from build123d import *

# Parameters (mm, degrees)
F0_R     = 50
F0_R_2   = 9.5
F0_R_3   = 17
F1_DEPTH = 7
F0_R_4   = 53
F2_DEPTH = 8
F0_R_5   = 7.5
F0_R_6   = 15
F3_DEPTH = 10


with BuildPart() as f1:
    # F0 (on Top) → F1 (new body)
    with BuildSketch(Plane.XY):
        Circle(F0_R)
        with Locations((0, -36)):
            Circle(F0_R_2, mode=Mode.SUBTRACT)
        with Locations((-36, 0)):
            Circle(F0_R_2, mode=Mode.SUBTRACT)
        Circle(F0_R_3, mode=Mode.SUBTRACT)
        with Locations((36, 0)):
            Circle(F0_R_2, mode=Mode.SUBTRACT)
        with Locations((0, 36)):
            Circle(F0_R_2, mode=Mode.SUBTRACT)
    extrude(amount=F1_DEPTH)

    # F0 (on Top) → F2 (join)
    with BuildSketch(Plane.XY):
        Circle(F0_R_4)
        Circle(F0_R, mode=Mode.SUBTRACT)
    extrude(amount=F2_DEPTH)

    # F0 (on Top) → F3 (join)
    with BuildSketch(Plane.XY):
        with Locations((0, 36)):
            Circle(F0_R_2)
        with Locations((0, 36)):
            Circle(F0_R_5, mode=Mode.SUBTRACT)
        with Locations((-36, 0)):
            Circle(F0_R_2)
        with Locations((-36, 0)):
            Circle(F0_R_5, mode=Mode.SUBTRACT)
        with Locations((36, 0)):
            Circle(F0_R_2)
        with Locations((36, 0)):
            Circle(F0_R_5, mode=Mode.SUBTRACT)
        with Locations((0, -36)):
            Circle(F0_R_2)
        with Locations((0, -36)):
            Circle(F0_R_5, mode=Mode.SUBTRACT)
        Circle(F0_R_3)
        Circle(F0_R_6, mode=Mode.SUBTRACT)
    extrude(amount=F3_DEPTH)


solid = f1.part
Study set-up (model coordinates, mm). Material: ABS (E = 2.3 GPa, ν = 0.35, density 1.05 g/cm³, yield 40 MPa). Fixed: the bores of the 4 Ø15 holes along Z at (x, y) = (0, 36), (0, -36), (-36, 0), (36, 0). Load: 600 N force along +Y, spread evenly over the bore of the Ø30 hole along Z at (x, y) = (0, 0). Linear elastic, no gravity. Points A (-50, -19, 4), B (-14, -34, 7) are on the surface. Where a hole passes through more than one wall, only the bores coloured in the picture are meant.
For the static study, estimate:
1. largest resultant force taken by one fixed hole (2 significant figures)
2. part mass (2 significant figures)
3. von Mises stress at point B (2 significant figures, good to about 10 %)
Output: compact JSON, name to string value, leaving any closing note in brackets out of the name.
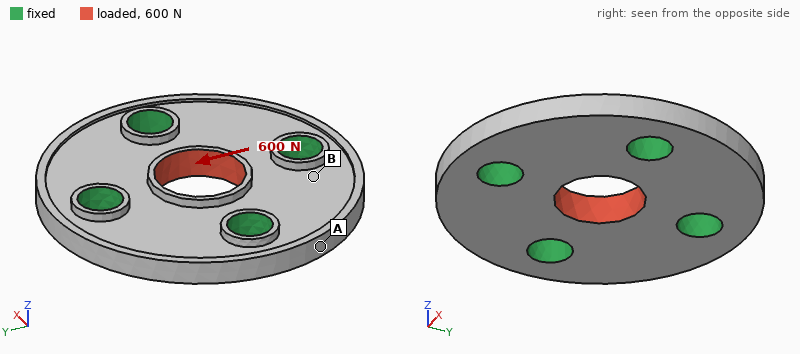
{"largest resultant force taken by one fixed hole": "190 N", "part mass": "57 g", "von Mises stress at point B": "0.41 MPa"}
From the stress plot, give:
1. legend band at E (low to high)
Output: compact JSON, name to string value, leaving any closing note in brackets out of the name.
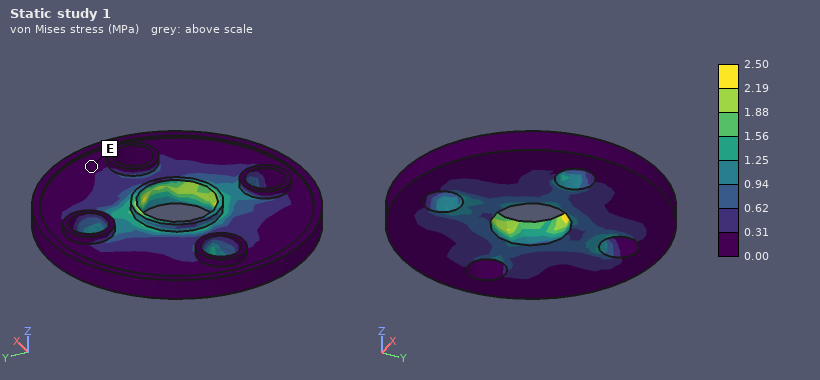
{"legend band at E": "0.00 to 0.31 MPa"}
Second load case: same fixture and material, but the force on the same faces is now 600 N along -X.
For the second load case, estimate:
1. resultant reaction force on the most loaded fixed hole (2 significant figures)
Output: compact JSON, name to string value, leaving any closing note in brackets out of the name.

{"resultant reaction force on the most loaded fixed hole": "190 N"}
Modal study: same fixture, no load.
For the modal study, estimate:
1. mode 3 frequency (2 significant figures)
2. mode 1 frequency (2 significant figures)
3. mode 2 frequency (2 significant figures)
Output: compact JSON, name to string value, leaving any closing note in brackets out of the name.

{"mode 3 frequency": "3100 Hz", "mode 1 frequency": "3100 Hz", "mode 2 frequency": "3100 Hz"}
